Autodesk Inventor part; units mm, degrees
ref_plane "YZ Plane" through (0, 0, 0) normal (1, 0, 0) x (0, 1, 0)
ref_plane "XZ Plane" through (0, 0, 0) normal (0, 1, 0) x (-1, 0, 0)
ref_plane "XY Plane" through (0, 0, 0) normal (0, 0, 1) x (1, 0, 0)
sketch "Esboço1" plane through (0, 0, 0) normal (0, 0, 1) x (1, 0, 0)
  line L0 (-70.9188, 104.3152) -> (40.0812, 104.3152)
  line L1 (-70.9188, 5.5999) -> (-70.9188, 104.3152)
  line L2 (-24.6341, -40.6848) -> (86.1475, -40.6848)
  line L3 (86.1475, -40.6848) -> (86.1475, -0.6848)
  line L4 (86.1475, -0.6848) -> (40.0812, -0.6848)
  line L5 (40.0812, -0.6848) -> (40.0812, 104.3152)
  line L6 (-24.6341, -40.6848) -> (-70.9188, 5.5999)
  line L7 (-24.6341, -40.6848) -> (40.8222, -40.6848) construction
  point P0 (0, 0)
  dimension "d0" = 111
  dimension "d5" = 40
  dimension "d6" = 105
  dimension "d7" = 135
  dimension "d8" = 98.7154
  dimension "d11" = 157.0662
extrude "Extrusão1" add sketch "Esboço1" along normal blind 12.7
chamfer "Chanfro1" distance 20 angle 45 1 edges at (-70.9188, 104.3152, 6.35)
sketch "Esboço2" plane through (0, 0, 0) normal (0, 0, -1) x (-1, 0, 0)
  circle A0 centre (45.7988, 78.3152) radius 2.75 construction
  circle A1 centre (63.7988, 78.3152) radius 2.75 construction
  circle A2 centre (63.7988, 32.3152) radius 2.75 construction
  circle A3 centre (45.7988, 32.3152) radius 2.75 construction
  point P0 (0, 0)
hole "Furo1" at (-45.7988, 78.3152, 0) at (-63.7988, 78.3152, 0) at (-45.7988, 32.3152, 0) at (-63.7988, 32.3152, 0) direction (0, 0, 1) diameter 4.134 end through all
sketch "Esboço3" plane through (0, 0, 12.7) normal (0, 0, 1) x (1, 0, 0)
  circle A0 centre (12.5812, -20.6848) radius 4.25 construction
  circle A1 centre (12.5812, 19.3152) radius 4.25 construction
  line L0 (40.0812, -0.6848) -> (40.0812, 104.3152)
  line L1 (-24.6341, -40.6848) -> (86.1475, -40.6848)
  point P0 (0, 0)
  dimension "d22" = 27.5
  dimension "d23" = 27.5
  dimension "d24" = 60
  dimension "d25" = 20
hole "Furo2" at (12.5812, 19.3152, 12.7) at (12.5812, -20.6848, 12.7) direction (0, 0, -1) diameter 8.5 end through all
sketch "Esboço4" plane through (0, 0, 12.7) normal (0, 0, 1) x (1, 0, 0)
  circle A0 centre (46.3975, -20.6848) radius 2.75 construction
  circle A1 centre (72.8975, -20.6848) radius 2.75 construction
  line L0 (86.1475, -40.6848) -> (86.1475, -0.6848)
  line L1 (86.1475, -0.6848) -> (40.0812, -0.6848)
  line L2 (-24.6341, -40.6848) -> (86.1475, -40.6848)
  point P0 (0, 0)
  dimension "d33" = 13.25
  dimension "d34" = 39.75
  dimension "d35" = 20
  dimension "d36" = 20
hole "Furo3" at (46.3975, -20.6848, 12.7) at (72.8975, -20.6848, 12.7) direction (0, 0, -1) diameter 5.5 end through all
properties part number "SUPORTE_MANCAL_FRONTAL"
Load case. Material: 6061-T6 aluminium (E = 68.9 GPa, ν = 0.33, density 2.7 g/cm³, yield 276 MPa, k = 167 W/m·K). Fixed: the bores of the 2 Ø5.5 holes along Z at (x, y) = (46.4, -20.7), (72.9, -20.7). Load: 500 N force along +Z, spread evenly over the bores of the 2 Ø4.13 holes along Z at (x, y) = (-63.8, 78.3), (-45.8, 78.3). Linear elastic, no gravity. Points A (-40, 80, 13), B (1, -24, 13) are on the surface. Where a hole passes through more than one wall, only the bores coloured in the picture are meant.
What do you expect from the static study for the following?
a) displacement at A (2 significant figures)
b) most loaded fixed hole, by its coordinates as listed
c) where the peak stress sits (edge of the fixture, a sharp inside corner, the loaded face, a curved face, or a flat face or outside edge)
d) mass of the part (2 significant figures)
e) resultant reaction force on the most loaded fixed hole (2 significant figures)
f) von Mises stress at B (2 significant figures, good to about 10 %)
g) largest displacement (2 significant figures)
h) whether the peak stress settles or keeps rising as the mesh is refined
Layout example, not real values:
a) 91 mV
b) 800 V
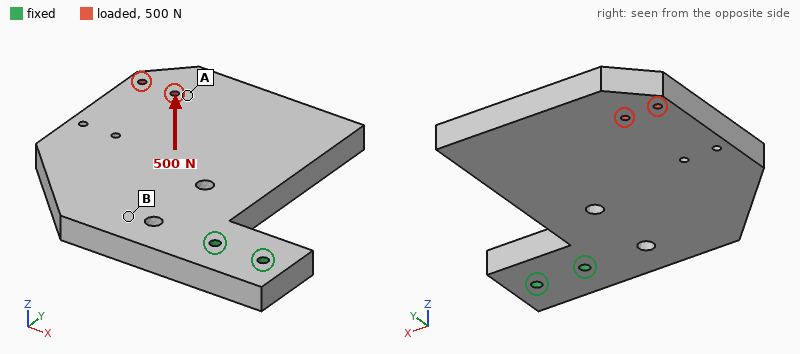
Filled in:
a) 0.72 mm
b) (46.4, -20.7)
c) edge of the fixture
d) 560 g
e) 1.3 kN
f) 27 MPa
g) 0.90 mm
h) keeps rising
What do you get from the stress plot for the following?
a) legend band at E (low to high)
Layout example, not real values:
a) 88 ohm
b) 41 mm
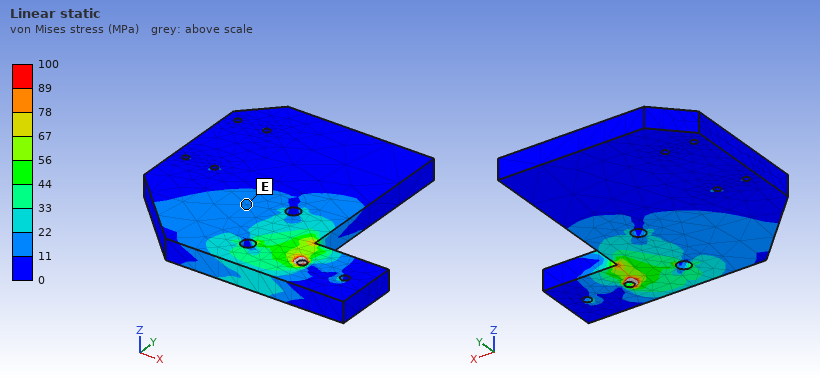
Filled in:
a) 11 to 22 MPa
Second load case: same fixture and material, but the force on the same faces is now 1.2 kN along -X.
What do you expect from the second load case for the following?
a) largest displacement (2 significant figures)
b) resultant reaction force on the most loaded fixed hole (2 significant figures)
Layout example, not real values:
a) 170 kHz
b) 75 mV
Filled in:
a) 0.20 mm
b) 3.7 kN
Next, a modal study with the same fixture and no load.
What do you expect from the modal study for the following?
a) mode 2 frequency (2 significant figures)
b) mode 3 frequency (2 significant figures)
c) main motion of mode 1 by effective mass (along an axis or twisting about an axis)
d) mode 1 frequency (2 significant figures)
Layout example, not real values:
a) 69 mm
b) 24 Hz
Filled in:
a) 730 Hz
b) 750 Hz
c) along Z
d) 310 Hz
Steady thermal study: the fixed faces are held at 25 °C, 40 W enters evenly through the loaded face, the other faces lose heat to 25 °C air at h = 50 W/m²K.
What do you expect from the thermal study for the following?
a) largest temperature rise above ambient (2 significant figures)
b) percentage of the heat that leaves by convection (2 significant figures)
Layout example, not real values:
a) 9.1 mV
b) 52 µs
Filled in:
a) 27 K
b) 58 %
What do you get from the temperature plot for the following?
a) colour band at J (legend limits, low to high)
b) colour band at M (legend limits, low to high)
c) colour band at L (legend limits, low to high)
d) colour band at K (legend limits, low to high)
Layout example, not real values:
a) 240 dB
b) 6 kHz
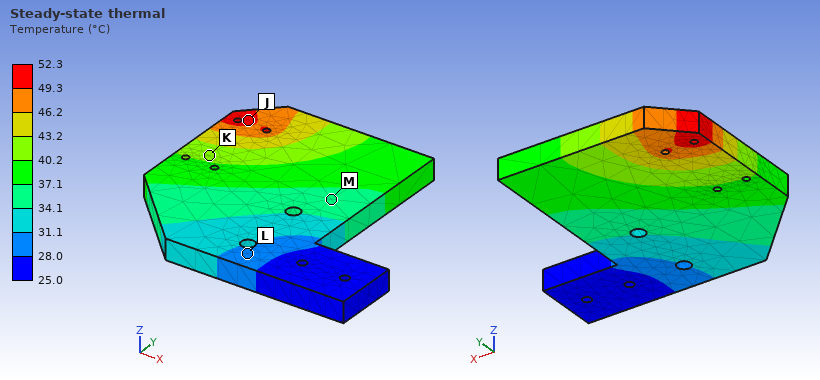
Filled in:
a) 49.3 to 52.3 °C
b) 34.1 to 37.1 °C
c) 28.0 to 31.1 °C
d) 40.2 to 43.2 °C
